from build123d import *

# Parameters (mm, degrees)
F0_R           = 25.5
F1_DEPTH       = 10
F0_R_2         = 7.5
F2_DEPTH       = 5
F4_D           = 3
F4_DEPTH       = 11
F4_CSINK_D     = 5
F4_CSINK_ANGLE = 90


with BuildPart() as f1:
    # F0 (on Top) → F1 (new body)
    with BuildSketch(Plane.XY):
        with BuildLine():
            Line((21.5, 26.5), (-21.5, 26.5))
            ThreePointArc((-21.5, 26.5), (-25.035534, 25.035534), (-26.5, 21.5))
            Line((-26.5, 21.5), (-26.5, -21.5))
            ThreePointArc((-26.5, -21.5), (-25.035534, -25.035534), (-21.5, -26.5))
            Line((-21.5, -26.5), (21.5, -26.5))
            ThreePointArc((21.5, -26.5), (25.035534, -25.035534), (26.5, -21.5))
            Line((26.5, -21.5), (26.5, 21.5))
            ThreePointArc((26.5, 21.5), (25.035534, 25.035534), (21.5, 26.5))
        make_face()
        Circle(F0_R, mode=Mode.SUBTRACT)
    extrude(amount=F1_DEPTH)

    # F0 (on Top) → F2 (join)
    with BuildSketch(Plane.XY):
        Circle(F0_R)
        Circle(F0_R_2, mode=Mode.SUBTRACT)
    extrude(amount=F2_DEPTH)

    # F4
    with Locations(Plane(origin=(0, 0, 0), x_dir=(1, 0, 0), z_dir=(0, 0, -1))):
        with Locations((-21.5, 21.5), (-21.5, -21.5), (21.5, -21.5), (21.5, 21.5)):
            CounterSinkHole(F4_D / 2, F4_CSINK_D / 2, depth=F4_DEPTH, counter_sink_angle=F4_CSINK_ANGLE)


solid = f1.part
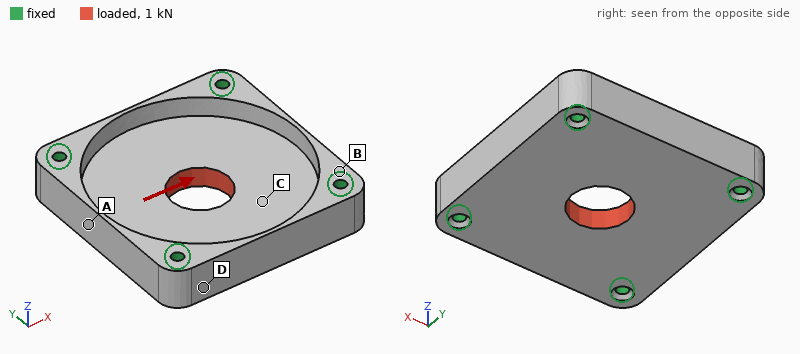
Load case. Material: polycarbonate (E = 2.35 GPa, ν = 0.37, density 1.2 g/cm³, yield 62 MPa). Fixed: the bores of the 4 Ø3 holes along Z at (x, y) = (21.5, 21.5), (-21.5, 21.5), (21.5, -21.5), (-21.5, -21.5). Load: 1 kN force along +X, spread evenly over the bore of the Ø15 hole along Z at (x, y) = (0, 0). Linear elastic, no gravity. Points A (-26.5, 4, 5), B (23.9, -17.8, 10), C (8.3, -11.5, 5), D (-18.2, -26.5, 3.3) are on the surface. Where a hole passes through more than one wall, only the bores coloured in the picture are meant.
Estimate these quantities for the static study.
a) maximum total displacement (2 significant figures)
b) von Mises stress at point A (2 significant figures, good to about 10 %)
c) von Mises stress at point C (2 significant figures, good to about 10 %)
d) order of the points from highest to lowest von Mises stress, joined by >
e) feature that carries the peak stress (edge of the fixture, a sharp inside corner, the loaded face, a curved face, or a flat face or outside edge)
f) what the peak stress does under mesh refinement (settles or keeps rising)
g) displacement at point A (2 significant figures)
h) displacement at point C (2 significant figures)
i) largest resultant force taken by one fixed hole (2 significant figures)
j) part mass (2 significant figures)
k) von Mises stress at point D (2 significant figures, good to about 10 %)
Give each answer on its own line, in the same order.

60 µm
2.7 MPa
3.9 MPa
C > A > D > B
edge of the fixture
keeps rising
40 µm
35 µm
270 N
20 g
1.5 MPa
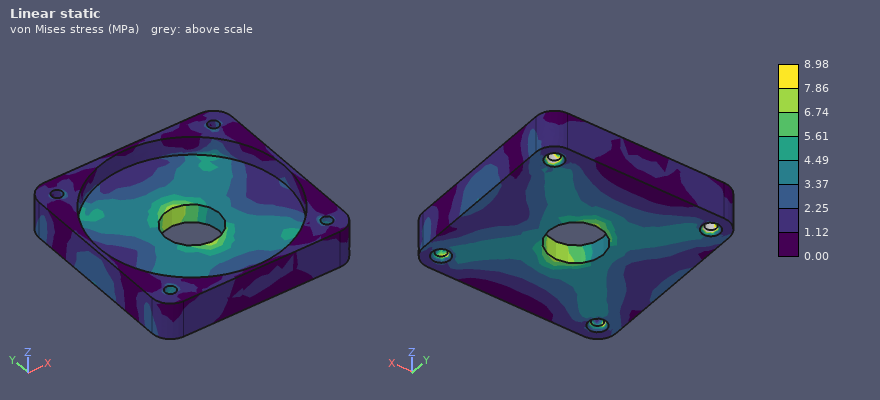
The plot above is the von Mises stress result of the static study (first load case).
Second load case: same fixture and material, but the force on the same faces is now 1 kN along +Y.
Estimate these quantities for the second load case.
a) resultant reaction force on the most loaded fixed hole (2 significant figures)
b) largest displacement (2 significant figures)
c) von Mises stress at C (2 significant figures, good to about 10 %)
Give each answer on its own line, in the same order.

270 N
60 µm
3.9 MPa
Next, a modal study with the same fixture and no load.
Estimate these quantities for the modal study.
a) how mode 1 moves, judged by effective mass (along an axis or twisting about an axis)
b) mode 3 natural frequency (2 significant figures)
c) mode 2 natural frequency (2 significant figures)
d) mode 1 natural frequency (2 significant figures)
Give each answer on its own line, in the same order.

along Z
5200 Hz
5200 Hz
3200 Hz
